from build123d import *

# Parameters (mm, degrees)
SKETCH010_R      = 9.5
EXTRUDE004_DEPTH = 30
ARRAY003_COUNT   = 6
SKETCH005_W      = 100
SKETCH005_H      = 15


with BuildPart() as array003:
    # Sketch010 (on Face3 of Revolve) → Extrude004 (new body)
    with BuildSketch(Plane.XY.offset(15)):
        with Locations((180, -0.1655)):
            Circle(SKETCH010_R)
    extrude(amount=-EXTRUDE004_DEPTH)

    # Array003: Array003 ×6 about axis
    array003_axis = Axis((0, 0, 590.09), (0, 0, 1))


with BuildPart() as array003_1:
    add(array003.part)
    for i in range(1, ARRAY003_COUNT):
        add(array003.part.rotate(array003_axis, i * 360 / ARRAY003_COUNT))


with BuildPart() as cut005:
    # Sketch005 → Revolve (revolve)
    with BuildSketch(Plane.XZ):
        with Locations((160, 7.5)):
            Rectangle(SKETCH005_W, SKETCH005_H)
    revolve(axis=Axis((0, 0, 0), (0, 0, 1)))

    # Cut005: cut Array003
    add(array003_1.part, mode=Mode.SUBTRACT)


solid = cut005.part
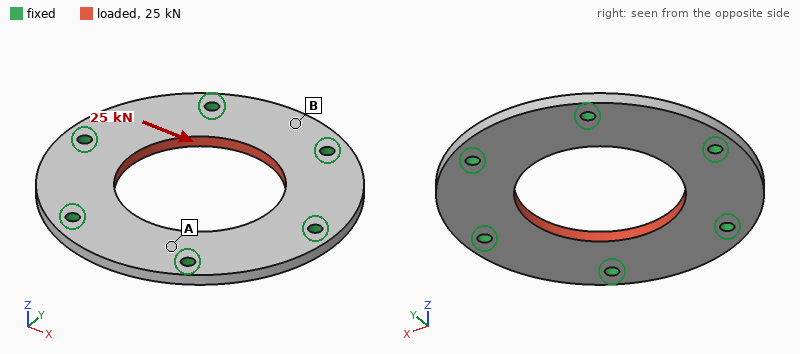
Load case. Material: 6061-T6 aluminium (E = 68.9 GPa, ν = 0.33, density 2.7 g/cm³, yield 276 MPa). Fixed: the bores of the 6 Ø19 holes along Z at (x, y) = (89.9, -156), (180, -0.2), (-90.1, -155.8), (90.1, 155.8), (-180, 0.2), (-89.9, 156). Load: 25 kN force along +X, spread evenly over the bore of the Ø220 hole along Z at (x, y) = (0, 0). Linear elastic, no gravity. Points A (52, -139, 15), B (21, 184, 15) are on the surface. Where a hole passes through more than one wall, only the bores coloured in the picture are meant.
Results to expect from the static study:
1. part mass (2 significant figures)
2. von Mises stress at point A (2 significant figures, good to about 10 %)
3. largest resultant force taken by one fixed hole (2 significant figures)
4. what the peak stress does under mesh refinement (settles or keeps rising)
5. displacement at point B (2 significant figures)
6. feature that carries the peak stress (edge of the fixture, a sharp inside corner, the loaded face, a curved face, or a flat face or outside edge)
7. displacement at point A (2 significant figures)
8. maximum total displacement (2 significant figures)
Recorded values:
4.0 kg
3.3 MPa
5.2 kN
keeps rising
1.2 µm
edge of the fixture
2.1 µm
6.4 µm
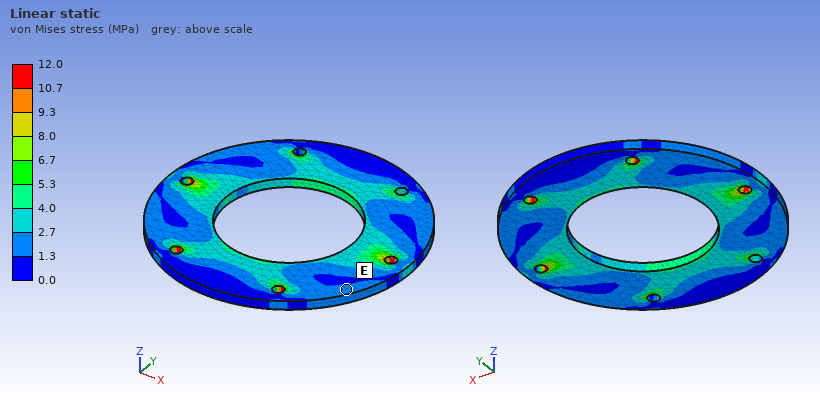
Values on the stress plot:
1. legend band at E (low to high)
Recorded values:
1.3 to 2.7 MPa
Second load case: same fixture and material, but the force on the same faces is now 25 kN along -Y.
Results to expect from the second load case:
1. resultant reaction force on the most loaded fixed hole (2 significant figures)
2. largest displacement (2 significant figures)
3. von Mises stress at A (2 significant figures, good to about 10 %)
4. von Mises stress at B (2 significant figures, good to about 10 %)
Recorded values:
4.8 kN
6.7 µm
3.1 MPa
1.6 MPa
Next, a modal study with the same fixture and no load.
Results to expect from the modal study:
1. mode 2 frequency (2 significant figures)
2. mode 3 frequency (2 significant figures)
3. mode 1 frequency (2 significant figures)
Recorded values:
2100 Hz
2200 Hz
2100 Hz
